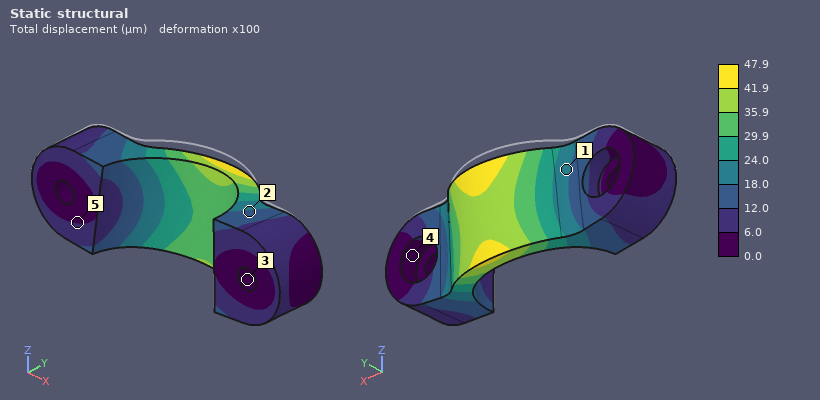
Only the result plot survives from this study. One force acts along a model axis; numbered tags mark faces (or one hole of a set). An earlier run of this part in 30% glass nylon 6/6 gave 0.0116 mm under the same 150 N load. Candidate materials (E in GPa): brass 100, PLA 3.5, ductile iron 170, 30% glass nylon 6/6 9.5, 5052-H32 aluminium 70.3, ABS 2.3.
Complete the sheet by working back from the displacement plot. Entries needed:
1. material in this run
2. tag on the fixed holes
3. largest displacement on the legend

ABS
3
47.9 µm
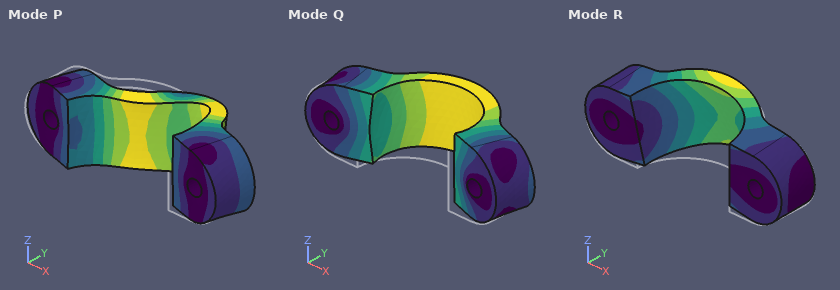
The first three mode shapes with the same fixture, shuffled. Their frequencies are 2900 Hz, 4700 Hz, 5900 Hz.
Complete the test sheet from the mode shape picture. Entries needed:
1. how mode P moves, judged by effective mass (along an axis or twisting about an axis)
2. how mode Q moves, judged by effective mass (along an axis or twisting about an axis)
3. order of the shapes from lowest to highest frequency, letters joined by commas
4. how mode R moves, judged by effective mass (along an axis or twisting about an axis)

along X
along Y
R, P, Q
along Z
